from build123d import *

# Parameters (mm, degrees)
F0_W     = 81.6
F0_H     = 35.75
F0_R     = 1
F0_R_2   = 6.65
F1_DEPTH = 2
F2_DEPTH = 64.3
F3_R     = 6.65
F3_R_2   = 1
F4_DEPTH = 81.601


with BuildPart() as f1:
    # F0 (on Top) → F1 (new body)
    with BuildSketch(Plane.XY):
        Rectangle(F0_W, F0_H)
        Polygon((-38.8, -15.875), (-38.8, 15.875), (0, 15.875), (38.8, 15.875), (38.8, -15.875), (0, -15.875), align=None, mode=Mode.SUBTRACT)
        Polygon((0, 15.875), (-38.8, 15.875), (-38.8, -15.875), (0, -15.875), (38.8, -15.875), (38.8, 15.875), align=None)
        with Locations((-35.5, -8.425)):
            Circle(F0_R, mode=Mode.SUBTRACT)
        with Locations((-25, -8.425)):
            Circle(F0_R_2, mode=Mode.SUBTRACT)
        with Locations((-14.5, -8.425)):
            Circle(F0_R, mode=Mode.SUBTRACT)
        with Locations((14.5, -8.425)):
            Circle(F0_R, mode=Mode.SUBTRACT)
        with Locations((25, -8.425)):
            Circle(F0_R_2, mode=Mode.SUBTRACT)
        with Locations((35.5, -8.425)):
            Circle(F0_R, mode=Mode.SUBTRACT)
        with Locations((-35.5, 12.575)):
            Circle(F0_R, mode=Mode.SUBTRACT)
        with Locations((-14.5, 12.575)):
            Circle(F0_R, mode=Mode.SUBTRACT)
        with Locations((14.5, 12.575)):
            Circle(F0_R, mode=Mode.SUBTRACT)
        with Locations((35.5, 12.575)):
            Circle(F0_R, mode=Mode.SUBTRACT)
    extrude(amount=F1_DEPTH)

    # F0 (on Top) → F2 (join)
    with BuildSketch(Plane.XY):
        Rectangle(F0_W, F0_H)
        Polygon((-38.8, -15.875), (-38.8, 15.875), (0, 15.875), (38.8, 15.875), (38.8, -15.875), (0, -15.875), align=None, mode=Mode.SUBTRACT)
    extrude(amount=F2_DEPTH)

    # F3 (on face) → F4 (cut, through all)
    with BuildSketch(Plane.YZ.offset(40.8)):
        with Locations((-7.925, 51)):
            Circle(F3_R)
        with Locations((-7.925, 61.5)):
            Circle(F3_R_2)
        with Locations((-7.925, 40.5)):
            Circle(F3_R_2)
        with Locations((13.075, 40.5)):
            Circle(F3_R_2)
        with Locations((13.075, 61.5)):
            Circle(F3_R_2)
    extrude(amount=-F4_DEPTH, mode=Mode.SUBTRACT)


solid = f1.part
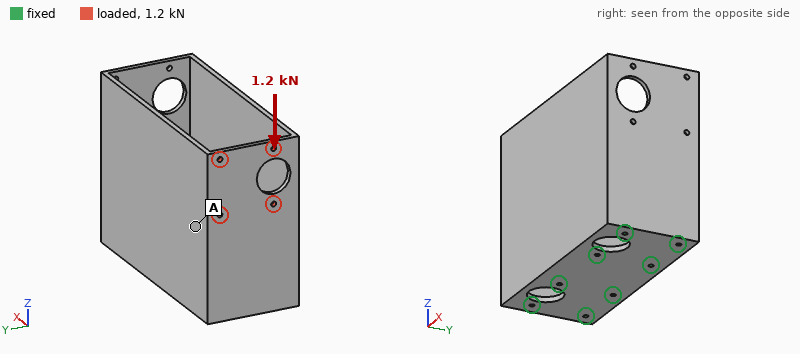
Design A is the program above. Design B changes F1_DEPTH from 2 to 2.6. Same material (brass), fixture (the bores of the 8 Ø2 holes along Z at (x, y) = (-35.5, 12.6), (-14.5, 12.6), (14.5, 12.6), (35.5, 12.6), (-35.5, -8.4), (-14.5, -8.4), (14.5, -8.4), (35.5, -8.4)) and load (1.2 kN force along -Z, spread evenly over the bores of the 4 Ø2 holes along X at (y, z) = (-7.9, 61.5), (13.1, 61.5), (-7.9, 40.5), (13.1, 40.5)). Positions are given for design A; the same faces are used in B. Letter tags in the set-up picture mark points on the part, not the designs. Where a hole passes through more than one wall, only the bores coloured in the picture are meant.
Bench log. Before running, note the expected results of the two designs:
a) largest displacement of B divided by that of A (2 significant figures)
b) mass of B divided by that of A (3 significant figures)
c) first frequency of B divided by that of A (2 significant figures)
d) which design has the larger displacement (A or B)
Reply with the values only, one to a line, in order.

0.76
1.04
1.0
A
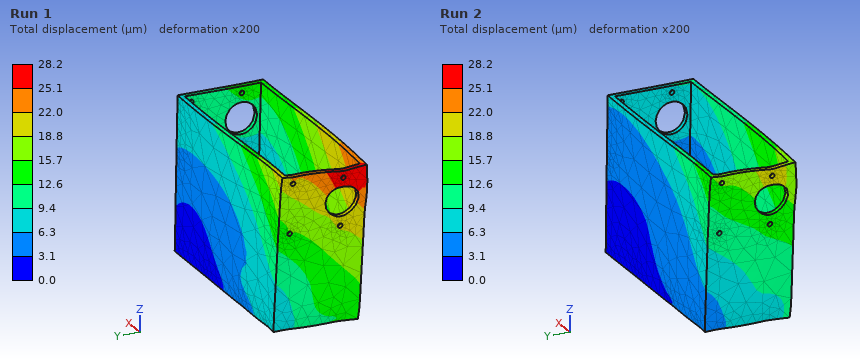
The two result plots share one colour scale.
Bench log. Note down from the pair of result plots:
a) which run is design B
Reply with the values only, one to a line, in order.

Run 2
